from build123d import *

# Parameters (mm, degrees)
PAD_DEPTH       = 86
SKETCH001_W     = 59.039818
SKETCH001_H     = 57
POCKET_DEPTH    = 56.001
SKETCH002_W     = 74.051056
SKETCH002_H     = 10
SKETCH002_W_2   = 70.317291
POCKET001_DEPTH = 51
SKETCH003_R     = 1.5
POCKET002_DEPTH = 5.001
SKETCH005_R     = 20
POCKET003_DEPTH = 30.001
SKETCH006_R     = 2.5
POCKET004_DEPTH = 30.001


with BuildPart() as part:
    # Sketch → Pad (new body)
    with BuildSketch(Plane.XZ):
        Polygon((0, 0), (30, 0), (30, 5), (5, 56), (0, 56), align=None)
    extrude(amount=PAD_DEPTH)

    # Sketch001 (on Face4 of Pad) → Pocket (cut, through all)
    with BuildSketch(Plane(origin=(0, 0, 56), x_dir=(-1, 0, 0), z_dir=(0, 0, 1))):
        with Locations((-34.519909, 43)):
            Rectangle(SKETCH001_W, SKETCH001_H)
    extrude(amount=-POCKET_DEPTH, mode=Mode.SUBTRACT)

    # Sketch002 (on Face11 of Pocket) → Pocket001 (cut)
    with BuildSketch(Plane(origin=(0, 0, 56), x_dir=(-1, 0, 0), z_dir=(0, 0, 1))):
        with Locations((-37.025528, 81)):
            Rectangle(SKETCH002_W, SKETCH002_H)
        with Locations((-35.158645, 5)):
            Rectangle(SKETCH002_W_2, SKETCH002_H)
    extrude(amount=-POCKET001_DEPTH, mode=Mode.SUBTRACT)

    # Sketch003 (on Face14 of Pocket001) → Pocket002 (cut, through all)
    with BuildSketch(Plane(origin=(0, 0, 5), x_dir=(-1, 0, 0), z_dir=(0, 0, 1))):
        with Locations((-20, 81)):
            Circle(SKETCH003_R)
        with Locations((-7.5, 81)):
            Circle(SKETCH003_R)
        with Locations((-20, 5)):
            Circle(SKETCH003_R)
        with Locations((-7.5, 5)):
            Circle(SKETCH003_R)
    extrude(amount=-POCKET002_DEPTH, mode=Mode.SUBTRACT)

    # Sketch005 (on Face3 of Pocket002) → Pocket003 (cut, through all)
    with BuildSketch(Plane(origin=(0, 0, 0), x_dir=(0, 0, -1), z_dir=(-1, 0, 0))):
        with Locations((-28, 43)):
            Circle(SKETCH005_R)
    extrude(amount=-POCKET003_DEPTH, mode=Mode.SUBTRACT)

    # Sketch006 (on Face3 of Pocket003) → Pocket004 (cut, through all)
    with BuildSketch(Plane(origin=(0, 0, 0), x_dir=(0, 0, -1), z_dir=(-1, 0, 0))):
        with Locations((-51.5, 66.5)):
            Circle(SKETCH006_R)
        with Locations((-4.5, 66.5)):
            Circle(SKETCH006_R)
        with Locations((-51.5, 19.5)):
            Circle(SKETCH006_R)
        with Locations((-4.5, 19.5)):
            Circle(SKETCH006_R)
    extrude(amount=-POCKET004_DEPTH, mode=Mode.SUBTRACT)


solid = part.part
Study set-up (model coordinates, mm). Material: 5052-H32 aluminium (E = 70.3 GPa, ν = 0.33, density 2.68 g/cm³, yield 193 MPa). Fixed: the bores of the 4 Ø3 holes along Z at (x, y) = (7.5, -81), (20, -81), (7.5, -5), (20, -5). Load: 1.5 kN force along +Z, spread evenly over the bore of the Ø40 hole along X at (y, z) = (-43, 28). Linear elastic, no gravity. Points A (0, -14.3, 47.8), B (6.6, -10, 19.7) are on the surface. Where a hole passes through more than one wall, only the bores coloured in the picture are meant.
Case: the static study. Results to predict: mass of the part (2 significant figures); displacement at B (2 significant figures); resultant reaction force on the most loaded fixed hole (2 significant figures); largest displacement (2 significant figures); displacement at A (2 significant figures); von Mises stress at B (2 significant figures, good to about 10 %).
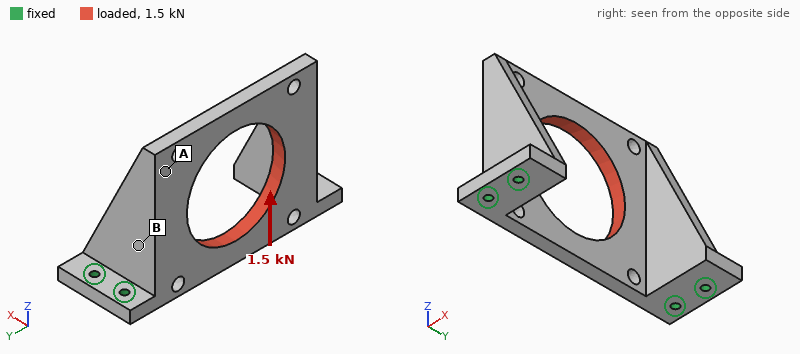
58 g
18 µm
920 N
56 µm
47 µm
13 MPa
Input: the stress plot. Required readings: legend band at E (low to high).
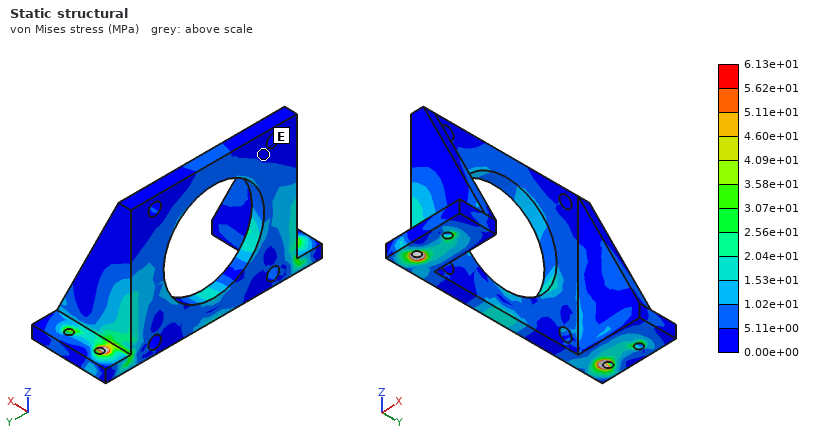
0.00e+00 to 5.11e+00 MPa
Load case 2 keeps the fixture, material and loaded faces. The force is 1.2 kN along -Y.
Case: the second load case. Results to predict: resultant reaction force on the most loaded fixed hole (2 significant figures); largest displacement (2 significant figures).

820 N
46 µm
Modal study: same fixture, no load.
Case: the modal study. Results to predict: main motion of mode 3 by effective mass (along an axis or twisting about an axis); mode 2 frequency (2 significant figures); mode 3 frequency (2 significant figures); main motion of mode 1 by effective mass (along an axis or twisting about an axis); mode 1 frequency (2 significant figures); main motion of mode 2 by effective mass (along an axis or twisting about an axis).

along Y
3900 Hz
5400 Hz
along X
2800 Hz
along Y
